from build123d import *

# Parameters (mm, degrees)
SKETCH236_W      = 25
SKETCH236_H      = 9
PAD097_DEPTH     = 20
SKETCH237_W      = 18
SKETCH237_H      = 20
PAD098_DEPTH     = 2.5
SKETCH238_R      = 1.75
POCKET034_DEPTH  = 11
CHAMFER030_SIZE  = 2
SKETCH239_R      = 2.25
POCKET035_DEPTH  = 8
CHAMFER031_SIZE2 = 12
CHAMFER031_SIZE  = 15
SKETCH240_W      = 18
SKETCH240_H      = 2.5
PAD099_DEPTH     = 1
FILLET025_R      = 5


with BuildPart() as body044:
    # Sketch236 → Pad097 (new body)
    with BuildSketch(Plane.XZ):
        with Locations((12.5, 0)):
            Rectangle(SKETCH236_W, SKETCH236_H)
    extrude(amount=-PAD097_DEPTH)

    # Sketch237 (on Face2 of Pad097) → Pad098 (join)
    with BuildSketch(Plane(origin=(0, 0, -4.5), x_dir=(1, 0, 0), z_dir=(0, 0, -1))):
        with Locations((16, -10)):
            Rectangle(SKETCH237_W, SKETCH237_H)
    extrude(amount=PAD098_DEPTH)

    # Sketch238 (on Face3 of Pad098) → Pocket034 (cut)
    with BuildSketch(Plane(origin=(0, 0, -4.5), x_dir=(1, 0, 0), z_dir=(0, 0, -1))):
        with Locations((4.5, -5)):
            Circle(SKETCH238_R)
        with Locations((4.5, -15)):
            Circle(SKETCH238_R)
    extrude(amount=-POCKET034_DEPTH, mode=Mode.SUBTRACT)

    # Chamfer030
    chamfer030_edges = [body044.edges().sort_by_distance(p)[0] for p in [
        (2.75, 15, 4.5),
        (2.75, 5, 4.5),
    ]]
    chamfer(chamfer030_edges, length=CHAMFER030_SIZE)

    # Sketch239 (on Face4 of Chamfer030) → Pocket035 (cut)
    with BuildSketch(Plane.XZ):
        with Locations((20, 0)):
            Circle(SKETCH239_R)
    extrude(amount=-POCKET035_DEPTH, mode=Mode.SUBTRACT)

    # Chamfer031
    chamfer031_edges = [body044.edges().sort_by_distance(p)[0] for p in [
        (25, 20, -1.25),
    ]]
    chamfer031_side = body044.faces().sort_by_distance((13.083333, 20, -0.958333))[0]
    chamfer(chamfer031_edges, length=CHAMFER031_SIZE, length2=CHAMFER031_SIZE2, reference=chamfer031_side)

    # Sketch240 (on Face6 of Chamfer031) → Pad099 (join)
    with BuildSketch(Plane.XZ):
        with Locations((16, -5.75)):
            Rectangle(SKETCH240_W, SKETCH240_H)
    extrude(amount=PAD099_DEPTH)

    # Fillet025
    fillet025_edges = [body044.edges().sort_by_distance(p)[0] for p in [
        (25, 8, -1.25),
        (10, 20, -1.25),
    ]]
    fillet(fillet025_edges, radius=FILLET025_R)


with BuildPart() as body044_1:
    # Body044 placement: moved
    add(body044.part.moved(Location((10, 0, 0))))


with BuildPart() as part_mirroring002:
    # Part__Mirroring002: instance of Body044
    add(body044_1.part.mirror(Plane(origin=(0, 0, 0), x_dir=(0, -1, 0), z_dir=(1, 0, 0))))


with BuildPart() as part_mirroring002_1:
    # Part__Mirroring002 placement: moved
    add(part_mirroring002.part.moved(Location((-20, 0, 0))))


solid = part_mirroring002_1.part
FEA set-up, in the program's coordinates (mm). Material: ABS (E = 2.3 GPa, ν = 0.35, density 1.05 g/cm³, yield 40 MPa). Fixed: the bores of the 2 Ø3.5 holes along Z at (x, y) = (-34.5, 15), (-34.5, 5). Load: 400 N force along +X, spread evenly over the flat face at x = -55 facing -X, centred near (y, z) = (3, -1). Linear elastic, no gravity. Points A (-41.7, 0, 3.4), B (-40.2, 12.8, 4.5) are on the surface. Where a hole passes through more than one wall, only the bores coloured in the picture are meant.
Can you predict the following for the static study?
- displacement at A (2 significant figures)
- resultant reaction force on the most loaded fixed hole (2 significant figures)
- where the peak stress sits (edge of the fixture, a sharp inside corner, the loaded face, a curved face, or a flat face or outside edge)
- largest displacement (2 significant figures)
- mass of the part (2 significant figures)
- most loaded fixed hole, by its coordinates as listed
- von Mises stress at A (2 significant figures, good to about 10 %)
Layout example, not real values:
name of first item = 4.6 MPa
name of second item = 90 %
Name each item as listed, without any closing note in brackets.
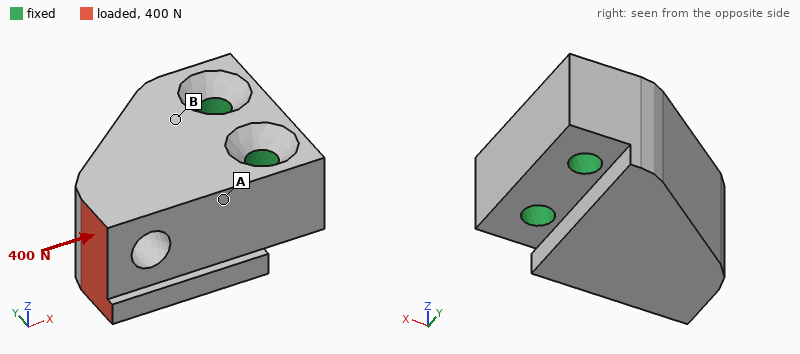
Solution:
displacement at A = 0.028 mm
resultant reaction force on the most loaded fixed hole = 450 N
where the peak stress sits = a curved face
largest displacement = 0.12 mm
mass of the part = 4.2 g
most loaded fixed hole, by its coordinates as listed = (-34.5, 5)
von Mises stress at A = 6.0 MPa
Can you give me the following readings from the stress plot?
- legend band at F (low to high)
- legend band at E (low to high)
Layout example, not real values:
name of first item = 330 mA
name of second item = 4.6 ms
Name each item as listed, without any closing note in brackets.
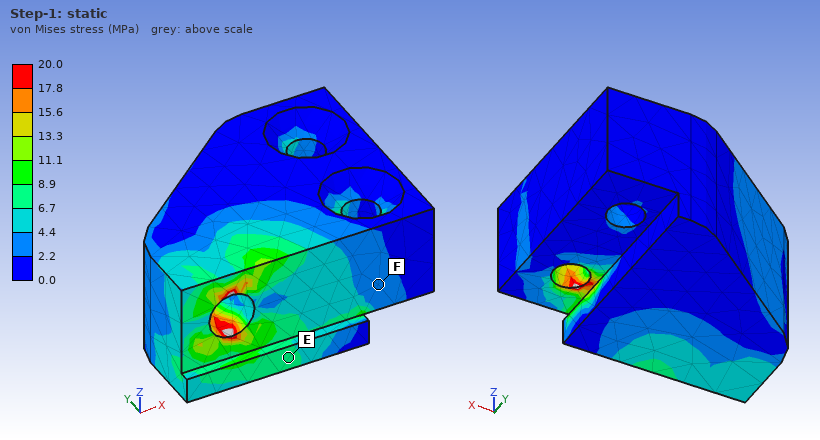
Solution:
legend band at F = 2.2 to 4.4 MPa
legend band at E = 6.7 to 8.9 MPa
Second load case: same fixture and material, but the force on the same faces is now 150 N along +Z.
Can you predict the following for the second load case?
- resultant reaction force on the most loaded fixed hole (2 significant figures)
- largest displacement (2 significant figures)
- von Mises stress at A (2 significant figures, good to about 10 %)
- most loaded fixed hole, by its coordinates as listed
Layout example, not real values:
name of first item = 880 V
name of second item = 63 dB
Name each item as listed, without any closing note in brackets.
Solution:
resultant reaction force on the most loaded fixed hole = 140 N
largest displacement = 0.28 mm
von Mises stress at A = 4.7 MPa
most loaded fixed hole, by its coordinates as listed = (-34.5, 5)
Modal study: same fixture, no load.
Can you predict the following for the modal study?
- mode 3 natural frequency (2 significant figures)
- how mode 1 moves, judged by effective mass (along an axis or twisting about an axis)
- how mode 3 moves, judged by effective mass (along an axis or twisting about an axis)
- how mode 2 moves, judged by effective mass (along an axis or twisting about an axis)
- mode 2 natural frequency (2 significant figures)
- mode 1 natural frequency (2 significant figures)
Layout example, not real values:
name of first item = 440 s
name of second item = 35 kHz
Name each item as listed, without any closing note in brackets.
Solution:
mode 3 natural frequency = 12 kHz
how mode 1 moves, judged by effective mass = along Z
how mode 3 moves, judged by effective mass = twisting about X
how mode 2 moves, judged by effective mass = along Y
mode 2 natural frequency = 8000 Hz
mode 1 natural frequency = 4800 Hz
